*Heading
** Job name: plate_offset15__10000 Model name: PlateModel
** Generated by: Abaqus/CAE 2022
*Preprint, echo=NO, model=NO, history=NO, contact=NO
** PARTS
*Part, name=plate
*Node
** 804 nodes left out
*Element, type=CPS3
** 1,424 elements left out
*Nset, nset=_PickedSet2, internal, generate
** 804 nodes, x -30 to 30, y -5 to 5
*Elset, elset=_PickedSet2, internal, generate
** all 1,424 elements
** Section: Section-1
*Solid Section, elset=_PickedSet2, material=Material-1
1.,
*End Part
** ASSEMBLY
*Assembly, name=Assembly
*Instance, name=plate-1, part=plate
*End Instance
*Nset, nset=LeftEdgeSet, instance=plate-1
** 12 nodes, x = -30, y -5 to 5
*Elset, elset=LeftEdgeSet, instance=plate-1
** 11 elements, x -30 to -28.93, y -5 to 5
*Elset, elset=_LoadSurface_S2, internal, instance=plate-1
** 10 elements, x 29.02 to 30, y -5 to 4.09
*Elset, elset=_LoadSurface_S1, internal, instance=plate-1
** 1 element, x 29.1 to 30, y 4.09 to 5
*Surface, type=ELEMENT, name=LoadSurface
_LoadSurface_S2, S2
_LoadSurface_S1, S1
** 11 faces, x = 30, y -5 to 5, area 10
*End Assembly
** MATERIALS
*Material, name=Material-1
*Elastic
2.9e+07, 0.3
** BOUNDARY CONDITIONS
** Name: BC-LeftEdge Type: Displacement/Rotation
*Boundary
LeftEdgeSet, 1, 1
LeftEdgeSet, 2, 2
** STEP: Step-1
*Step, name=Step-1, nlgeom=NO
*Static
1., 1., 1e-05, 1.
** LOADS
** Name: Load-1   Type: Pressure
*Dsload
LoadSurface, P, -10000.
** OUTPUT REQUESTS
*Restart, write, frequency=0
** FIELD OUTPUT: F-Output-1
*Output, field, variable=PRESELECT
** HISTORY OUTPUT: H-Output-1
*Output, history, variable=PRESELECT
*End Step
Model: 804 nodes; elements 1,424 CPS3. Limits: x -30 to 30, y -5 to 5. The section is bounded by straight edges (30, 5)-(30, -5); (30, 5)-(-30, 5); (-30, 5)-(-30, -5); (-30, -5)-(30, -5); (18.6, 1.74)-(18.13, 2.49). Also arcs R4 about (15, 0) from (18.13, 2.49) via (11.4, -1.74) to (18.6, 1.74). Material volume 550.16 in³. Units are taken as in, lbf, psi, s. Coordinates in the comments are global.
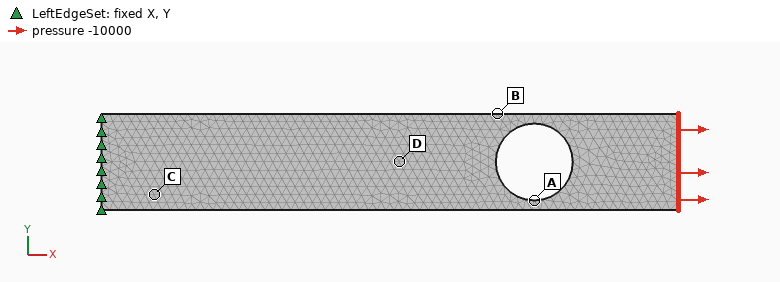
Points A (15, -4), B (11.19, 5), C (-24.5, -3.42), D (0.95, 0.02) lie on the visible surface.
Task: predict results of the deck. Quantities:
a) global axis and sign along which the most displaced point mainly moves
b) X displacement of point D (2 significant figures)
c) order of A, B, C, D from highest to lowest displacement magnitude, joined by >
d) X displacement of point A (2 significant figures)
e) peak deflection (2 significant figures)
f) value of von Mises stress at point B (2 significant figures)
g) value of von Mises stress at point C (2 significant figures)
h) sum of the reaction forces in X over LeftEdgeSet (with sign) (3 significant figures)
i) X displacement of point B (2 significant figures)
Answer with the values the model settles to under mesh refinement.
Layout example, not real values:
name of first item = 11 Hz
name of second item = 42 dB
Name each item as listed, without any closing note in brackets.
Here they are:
global axis and sign along which the most displaced point mainly moves = +X
X displacement of point D = 0.011 in
order of A, B, C, D from highest to lowest displacement magnitude, joined by > = A > B > D > C
X displacement of point A = 0.022 in
peak deflection = 0.034 in
value of von Mises stress at point B = 45000 psi
value of von Mises stress at point C = 9900 psi
sum of the reaction forces in X over LeftEdgeSet (with sign) = -1.00e+05 lbf
X displacement of point B = 0.018 in
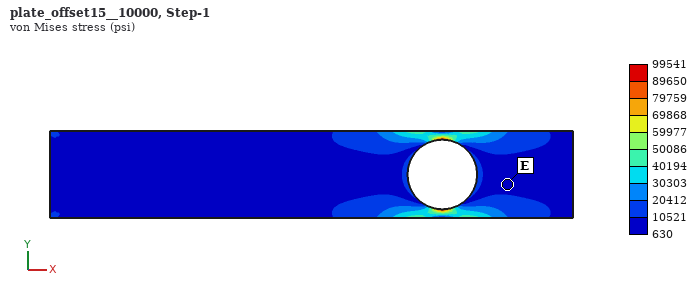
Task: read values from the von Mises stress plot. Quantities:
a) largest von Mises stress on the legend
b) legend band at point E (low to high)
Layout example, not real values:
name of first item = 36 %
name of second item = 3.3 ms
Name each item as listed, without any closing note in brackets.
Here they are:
largest von Mises stress on the legend = 99541 psi
legend band at point E = 630 to 10521 psi
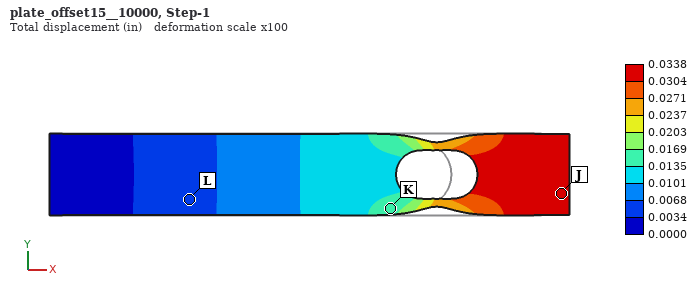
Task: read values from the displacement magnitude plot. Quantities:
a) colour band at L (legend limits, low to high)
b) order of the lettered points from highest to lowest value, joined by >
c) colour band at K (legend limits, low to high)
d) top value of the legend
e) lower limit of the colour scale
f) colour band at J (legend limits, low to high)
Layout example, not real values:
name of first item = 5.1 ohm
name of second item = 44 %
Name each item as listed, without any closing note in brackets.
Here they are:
colour band at L = 0.0034 to 0.0068 in
order of the lettered points from highest to lowest value, joined by > = J > K > L
colour band at K = 0.0135 to 0.0169 in
top value of the legend = 0.0338 in
lower limit of the colour scale = 0.0000 in
colour band at J = 0.0304 to 0.0338 in
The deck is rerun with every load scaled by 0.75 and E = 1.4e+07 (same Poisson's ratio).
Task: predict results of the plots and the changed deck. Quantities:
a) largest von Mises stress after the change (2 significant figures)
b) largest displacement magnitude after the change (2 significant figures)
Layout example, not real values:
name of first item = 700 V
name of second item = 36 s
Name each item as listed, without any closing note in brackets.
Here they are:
largest von Mises stress after the change = 75000 psi
largest displacement magnitude after the change = 0.053 in
